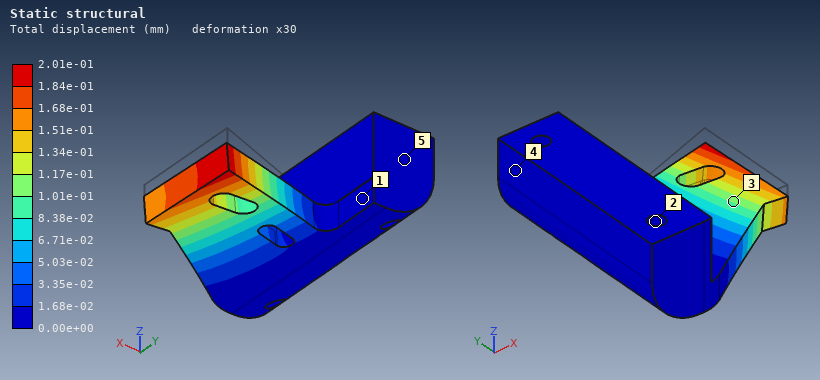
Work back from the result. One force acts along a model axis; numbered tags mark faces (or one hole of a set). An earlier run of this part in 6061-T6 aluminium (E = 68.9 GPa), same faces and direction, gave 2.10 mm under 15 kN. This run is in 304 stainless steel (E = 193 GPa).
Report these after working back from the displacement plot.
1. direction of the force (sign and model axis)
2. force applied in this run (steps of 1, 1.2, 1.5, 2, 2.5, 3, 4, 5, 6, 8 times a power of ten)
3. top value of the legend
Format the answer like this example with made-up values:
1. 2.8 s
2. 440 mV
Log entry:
1. -Z
2. 4 kN
3. 2.01e-01 mm
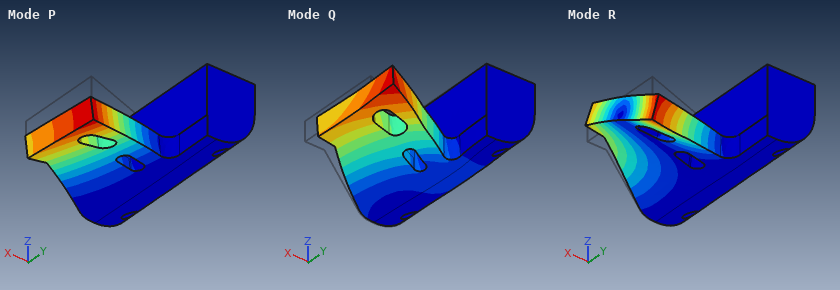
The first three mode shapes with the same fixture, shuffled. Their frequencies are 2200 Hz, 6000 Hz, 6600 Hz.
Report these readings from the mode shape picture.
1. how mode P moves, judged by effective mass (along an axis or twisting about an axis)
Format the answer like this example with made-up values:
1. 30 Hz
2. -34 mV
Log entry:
1. along Z
